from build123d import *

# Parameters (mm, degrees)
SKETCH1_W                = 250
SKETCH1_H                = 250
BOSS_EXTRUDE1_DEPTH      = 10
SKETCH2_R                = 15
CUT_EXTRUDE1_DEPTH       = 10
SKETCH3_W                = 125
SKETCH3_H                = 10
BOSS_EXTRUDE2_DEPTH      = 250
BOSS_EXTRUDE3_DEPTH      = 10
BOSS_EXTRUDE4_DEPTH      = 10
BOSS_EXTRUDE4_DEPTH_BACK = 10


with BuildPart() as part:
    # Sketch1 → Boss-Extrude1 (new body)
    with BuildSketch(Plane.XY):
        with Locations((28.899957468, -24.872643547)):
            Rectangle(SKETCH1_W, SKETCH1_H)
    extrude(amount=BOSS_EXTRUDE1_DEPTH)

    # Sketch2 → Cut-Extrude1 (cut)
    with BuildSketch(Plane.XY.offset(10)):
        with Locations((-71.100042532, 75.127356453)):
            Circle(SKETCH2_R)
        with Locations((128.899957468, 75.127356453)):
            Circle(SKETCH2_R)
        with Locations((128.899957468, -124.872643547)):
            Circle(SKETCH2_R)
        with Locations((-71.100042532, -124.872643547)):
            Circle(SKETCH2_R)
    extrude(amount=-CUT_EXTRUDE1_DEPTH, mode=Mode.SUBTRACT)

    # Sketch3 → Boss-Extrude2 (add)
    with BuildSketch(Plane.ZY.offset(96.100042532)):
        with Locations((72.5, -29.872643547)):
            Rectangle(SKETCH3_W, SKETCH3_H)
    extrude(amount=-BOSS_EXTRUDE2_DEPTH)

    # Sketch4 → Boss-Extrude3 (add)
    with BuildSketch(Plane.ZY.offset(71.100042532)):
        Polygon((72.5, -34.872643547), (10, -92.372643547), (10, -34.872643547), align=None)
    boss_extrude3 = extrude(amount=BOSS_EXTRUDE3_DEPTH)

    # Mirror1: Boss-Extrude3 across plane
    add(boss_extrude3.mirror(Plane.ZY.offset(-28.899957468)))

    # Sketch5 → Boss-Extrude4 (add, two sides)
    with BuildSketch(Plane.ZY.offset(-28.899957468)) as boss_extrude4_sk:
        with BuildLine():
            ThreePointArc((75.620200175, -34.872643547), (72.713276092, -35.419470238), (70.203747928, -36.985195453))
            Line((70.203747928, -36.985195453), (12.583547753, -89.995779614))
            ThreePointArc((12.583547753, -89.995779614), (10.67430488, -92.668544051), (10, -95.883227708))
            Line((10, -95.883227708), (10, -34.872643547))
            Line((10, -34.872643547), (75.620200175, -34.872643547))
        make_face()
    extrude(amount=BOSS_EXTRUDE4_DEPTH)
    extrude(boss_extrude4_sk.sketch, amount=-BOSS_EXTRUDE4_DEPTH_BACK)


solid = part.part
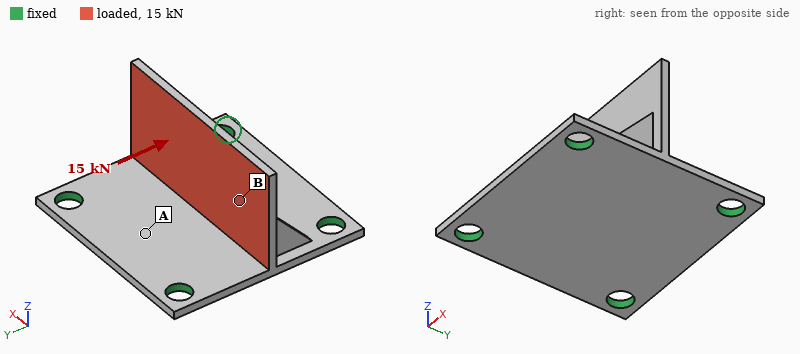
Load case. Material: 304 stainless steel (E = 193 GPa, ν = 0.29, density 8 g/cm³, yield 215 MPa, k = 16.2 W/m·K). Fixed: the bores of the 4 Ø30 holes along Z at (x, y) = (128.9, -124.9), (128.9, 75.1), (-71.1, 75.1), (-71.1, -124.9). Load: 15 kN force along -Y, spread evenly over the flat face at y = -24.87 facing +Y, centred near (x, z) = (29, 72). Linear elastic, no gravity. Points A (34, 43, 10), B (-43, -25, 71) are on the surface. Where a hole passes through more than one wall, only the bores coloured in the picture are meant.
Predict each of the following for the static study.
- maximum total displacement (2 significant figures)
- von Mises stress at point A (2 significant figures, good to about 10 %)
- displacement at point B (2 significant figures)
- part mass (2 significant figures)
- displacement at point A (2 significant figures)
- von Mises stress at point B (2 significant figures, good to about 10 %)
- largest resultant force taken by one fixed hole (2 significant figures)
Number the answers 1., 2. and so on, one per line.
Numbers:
1. 0.45 mm
2. 16 MPa
3. 0.18 mm
4. 7.8 kg
5. 0.067 mm
6. 43 MPa
7. 5.9 kN
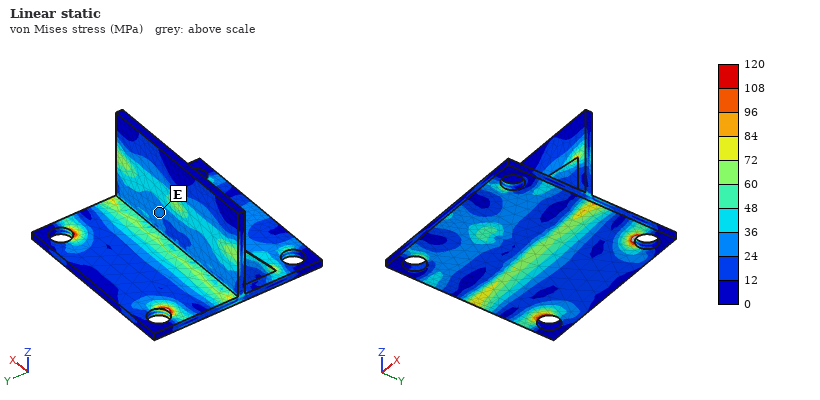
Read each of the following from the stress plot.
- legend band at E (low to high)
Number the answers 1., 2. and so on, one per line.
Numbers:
1. 24 to 36 MPa
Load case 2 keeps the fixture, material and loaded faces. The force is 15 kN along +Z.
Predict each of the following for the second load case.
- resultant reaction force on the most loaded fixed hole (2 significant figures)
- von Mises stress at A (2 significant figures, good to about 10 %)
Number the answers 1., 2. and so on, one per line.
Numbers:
1. 4.0 kN
2. 14 MPa
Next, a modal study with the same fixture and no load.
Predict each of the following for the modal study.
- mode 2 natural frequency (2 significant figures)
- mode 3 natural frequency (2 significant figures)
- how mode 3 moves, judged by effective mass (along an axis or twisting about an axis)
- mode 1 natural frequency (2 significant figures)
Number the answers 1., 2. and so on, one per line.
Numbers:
1. 800 Hz
2. 1100 Hz
3. along Z
4. 640 Hz
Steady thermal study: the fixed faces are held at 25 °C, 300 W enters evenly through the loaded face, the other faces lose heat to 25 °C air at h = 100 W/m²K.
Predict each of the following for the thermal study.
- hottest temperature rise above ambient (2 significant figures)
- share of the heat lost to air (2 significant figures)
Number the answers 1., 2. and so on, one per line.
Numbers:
1. 80 K
2. 99 %
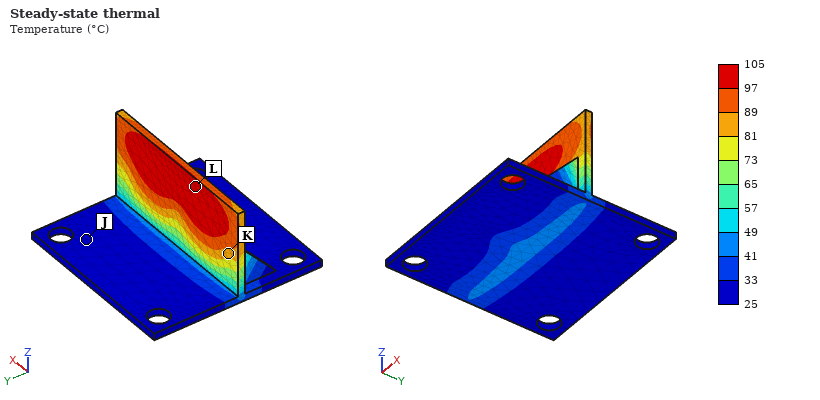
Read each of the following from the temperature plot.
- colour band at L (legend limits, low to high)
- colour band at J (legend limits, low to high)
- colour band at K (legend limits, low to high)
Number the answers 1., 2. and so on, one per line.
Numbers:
1. 97 to 105 °C
2. 25 to 33 °C
3. 81 to 89 °C
